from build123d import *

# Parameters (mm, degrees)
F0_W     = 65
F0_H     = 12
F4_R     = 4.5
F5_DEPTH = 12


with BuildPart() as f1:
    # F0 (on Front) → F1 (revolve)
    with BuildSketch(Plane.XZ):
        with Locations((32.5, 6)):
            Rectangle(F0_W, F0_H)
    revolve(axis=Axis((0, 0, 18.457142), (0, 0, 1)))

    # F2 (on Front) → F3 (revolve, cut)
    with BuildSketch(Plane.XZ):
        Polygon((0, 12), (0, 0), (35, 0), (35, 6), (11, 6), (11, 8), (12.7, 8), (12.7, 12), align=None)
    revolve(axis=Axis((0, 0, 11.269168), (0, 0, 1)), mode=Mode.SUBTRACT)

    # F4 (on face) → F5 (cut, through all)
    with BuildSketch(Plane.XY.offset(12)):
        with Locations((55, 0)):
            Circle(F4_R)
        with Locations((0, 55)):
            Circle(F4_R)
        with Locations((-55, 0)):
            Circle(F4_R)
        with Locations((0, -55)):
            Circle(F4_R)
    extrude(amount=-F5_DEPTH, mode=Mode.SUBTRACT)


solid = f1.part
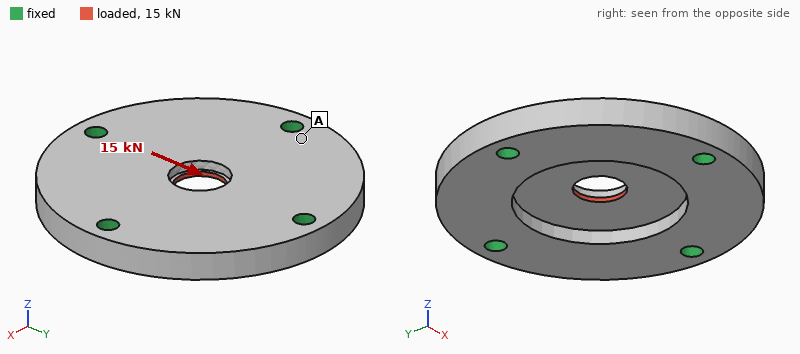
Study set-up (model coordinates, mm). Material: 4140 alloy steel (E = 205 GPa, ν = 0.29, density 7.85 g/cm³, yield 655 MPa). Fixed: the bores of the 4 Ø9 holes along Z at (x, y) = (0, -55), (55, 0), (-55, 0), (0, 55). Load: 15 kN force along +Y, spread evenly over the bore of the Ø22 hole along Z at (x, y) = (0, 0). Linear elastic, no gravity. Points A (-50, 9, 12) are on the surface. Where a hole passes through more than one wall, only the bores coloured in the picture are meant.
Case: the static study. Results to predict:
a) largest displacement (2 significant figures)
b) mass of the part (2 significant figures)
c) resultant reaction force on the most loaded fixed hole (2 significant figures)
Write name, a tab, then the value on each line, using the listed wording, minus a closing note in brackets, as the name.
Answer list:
largest displacement	9.2 µm
mass of the part	1.0 kg
resultant reaction force on the most loaded fixed hole	4.6 kN
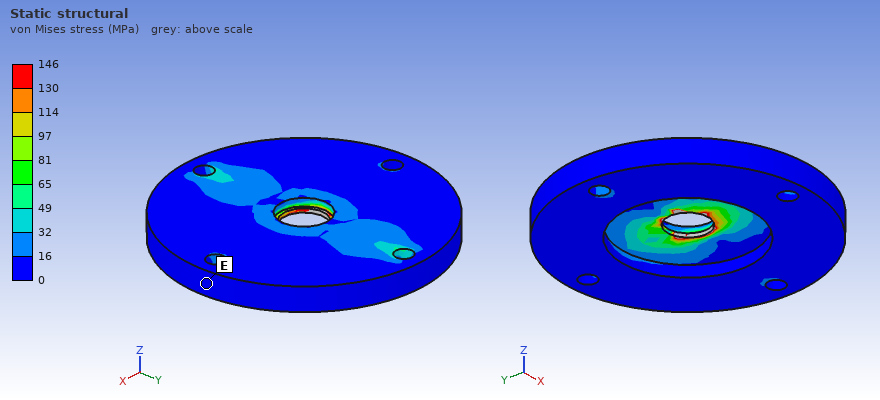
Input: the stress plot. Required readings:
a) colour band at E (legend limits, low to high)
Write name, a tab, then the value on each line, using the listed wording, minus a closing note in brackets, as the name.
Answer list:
colour band at E	0 to 16 MPa
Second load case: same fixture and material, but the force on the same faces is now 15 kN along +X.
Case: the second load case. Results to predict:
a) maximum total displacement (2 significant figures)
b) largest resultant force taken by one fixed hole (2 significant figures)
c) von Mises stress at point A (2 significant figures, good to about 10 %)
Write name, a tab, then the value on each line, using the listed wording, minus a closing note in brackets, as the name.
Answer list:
maximum total displacement	9.2 µm
largest resultant force taken by one fixed hole	4.6 kN
von Mises stress at point A	18 MPa
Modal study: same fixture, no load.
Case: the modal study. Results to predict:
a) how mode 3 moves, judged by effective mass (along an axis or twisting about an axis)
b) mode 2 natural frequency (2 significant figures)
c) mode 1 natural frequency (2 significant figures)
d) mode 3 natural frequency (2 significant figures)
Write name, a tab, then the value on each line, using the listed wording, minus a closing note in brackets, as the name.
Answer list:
how mode 3 moves, judged by effective mass	twisting about X
mode 2 natural frequency	7500 Hz
mode 1 natural frequency	7400 Hz
mode 3 natural frequency	8000 Hz
